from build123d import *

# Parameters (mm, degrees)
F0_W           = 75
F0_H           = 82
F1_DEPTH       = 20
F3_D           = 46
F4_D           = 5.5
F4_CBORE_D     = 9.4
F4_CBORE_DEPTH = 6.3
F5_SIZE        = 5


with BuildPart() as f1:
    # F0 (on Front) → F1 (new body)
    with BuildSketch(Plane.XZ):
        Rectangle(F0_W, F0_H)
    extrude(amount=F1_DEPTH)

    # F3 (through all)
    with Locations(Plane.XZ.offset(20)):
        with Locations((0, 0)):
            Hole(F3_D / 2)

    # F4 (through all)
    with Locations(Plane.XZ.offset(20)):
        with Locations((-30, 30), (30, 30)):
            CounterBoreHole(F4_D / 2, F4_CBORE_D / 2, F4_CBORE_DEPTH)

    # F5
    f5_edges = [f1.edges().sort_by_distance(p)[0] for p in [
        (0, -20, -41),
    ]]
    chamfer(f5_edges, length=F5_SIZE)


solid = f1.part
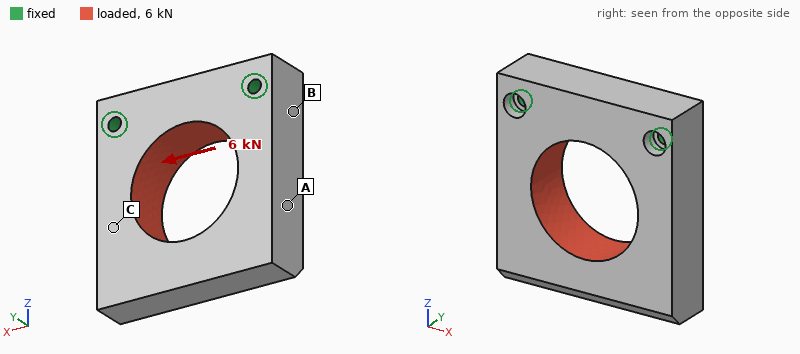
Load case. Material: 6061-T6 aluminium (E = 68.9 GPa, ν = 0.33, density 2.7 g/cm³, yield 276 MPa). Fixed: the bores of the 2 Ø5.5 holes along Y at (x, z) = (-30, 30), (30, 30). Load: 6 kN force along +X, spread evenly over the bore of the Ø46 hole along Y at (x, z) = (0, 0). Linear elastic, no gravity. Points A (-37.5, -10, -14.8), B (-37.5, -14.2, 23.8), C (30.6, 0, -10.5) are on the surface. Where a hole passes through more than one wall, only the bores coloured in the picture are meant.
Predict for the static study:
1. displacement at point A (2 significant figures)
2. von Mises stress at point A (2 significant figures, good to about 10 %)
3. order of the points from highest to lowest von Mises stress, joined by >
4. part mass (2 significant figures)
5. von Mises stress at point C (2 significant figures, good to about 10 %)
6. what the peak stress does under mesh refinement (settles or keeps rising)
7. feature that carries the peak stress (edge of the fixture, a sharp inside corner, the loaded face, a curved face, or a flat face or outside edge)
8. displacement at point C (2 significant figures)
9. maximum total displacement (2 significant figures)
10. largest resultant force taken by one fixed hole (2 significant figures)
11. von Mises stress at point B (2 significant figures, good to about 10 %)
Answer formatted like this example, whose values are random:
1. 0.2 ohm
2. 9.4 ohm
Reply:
1. 36 µm
2. 14 MPa
3. B > A > C
4. 240 g
5. 5.2 MPa
6. keeps rising
7. edge of the fixture
8. 34 µm
9. 45 µm
10. 4.0 kN
11. 22 MPa
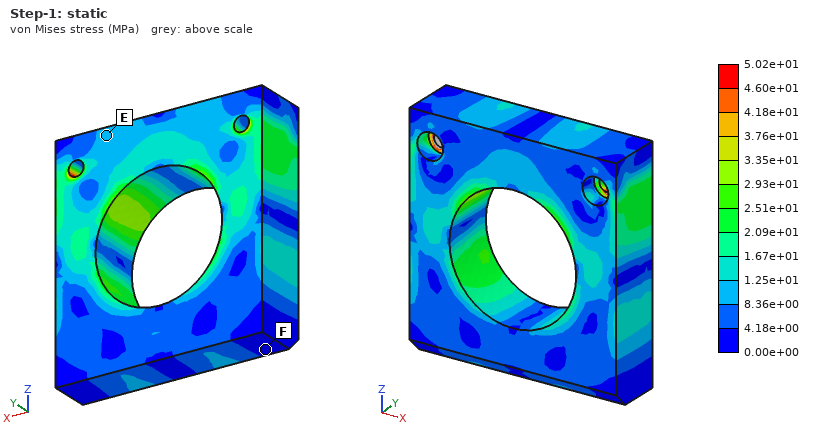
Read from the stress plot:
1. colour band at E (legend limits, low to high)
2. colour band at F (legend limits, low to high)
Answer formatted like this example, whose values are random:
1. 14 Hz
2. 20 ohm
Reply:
1. 8.36e+00 to 1.25e+01 MPa
2. 0.00e+00 to 4.18e+00 MPa
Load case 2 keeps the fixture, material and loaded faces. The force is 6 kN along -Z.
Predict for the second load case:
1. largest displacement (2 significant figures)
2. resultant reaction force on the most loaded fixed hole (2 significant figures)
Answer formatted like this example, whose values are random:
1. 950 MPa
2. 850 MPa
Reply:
1. 15 µm
2. 3.0 kN
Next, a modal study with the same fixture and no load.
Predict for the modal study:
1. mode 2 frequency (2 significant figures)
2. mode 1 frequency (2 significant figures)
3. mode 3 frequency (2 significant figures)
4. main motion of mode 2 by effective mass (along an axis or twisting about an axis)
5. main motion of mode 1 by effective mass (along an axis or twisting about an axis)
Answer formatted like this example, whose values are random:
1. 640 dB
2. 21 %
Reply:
1. 4100 Hz
2. 1900 Hz
3. 4500 Hz
4. along X
5. along Y
